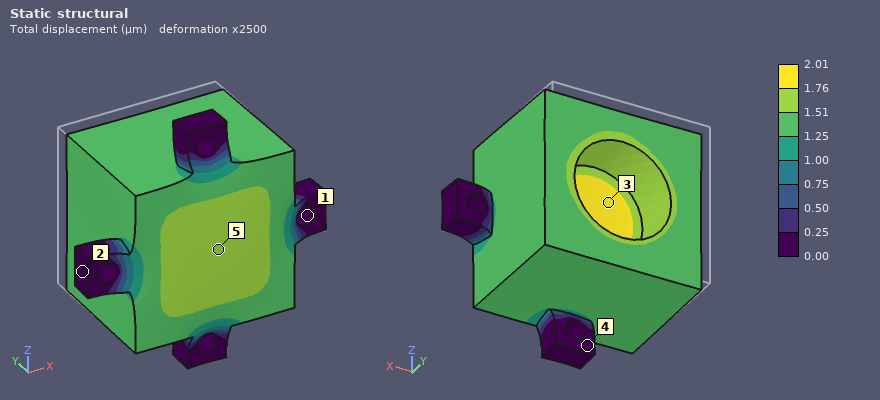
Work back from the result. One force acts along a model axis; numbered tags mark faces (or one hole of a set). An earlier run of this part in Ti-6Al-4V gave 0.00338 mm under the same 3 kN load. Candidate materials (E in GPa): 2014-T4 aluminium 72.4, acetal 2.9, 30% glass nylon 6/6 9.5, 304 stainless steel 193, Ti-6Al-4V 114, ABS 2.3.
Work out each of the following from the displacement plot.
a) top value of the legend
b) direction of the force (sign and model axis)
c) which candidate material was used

2.01 µm
-Y
304 stainless steel
